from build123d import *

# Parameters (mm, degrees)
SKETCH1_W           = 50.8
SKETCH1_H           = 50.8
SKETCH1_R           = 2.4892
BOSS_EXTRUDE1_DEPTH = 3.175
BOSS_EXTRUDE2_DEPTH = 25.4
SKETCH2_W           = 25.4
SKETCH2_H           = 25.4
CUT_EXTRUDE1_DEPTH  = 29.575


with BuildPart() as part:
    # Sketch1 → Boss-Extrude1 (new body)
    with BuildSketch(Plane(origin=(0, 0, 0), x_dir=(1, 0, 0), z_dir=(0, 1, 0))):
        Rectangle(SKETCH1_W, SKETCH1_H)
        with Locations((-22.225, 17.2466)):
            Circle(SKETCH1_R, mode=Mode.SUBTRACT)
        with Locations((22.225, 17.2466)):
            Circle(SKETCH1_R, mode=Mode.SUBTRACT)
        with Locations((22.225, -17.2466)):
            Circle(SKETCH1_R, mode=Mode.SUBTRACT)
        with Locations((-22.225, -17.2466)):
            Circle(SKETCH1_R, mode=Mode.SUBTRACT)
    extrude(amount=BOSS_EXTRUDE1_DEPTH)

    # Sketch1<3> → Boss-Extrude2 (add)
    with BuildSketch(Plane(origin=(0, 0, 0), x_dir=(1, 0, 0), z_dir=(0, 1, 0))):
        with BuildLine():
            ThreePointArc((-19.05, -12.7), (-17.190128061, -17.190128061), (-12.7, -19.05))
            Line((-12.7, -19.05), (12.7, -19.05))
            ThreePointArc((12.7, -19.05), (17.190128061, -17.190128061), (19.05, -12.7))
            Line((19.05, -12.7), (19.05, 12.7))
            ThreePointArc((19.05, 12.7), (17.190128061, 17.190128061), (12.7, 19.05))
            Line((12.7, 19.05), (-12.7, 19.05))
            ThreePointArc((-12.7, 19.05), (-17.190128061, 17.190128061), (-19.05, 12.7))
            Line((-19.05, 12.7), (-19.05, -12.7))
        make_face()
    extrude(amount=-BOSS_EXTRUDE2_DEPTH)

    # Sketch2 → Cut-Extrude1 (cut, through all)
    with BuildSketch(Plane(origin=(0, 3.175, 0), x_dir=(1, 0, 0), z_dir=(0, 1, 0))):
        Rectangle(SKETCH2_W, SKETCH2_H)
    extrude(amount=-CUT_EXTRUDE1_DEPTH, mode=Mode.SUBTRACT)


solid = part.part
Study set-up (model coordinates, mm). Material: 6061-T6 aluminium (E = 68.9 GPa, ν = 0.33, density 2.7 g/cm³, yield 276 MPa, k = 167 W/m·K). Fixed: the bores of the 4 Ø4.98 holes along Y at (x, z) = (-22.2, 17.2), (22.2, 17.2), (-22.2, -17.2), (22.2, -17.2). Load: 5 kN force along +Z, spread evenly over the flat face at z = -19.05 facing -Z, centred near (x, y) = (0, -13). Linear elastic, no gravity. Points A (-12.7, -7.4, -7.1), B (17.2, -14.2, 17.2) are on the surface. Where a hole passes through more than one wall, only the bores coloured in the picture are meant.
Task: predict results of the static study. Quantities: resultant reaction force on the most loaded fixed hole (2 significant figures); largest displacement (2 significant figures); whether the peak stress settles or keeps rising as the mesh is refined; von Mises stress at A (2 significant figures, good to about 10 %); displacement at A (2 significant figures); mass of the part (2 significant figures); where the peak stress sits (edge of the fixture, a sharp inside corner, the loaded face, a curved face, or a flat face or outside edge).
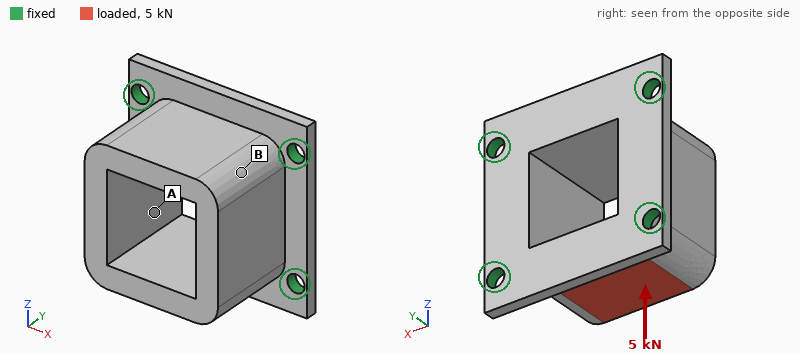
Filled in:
1.8 kN
68 µm
keeps rising
38 MPa
17 µm
69 g
edge of the fixture
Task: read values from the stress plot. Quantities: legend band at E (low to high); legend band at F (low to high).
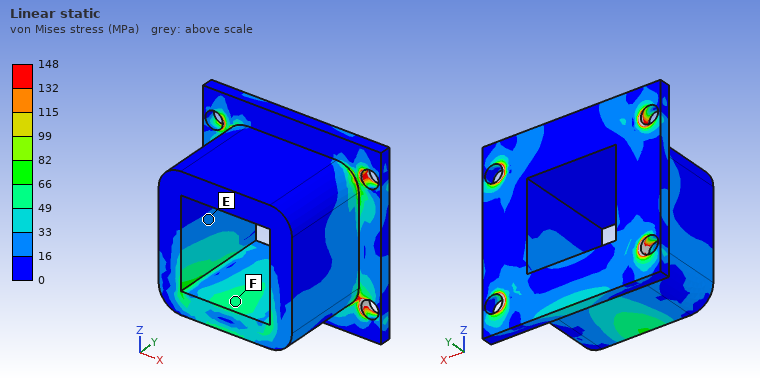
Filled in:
16 to 33 MPa
49 to 66 MPa
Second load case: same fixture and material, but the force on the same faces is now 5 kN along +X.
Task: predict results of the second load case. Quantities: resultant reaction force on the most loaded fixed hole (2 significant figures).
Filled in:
2.6 kN
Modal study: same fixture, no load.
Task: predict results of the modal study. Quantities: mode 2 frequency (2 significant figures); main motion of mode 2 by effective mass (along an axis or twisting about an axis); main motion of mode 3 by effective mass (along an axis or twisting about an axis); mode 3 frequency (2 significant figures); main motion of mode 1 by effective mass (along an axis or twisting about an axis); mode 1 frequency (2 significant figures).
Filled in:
11 kHz
along X
along Y
11 kHz
along Z
8700 Hz
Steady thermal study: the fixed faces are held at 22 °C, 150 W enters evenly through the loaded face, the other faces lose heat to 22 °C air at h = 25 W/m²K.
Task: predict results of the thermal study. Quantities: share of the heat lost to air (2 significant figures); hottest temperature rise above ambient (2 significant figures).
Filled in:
5.2 %
77 K
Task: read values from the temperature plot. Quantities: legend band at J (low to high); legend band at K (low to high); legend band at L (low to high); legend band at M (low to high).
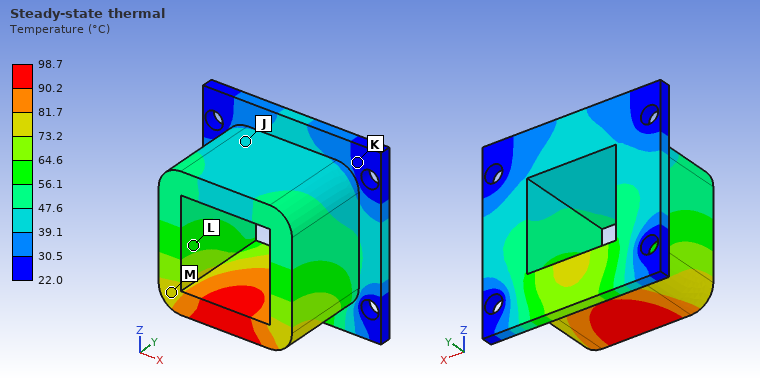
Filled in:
39.1 to 47.6 °C
22.0 to 30.5 °C
56.1 to 64.6 °C
73.2 to 81.7 °C
